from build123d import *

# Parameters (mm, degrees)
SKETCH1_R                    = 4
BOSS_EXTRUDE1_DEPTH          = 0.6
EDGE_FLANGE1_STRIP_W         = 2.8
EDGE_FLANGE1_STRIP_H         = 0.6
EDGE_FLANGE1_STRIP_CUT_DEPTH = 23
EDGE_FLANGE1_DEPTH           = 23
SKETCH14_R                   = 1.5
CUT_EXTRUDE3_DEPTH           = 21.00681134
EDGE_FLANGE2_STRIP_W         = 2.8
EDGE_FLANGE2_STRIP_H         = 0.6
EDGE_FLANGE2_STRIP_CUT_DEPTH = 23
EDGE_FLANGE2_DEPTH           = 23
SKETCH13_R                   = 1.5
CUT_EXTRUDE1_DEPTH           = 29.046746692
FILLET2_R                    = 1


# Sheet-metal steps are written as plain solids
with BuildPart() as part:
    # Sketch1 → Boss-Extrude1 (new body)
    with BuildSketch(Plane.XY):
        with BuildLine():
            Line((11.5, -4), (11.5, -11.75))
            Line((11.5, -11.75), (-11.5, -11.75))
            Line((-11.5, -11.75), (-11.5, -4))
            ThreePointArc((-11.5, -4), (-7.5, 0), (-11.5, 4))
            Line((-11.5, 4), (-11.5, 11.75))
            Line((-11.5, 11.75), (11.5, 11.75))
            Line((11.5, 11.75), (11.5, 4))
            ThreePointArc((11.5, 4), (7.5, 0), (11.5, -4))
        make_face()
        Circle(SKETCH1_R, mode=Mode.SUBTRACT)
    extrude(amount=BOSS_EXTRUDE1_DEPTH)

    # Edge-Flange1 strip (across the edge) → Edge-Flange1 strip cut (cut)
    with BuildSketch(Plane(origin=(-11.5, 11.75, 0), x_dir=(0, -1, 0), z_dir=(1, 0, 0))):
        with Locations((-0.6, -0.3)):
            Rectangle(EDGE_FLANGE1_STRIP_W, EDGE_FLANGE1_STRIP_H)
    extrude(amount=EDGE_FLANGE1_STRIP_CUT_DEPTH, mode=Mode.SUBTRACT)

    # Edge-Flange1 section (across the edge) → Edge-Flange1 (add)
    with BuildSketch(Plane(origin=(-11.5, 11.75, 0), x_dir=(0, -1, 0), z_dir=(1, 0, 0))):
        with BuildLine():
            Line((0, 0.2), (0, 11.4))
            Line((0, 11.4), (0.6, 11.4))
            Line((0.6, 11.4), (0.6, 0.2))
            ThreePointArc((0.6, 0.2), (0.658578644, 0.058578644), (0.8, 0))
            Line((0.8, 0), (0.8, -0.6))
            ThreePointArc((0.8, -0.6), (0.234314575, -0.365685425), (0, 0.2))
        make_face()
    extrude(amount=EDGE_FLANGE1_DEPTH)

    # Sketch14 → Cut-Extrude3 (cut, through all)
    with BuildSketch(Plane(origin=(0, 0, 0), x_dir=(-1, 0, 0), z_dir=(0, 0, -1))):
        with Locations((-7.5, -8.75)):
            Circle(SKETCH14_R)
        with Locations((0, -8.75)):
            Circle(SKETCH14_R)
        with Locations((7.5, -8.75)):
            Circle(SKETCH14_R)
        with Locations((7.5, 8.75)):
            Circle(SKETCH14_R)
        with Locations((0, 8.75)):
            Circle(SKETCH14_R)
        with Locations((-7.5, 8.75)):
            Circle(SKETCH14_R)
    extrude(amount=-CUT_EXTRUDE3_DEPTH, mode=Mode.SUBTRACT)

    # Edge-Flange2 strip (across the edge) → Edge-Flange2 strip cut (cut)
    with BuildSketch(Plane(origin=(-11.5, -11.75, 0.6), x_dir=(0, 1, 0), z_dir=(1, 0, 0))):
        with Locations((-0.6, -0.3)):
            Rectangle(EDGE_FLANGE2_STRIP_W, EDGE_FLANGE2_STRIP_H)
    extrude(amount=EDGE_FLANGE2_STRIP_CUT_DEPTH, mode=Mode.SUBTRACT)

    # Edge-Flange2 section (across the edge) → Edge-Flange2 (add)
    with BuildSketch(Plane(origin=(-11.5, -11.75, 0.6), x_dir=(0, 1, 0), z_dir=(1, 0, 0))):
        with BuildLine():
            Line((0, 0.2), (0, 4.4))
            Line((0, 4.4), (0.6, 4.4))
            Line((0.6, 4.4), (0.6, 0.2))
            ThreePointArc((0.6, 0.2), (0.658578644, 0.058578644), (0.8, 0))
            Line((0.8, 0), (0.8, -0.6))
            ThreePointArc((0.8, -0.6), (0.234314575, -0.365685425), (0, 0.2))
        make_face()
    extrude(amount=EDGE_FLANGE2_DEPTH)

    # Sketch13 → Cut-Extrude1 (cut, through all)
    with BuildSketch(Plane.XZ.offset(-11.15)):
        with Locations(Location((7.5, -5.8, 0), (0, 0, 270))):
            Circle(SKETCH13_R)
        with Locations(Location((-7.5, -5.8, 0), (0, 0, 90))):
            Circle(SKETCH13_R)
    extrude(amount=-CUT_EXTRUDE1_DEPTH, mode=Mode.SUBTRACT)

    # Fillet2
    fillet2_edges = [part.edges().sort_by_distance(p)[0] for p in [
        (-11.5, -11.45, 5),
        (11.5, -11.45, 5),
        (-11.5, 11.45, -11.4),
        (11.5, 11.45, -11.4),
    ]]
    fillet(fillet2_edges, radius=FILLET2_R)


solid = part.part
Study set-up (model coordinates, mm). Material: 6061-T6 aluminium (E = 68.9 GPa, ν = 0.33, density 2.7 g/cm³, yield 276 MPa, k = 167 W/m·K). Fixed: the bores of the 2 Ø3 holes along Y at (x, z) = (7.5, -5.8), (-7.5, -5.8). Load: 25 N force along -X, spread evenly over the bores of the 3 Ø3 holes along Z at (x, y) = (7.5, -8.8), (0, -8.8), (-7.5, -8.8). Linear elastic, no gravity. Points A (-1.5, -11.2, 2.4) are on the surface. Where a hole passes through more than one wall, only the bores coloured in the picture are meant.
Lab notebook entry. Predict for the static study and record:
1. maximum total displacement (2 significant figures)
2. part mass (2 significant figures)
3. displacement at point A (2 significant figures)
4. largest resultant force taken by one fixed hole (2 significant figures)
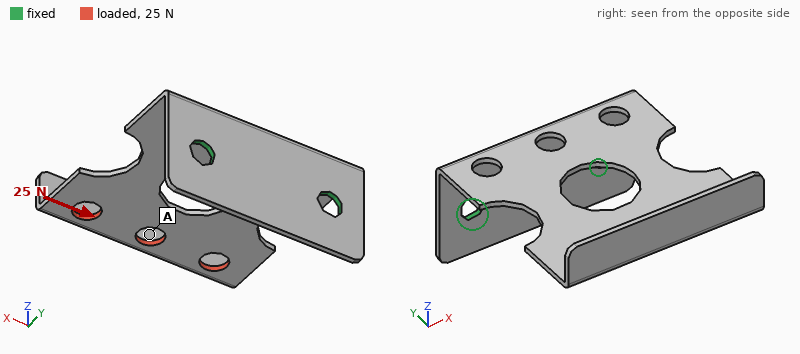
0.32 mm
1.2 g
0.21 mm
34 N
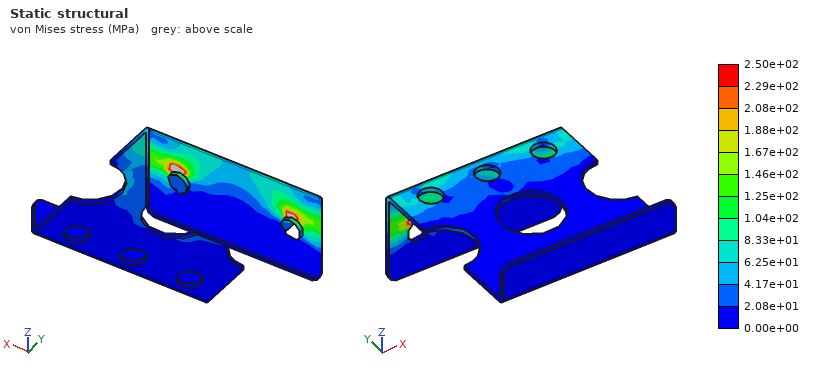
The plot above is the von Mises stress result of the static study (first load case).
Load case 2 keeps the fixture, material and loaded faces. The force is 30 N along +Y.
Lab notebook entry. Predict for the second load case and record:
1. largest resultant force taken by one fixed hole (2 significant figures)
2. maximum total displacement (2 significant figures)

15 N
0.34 mm
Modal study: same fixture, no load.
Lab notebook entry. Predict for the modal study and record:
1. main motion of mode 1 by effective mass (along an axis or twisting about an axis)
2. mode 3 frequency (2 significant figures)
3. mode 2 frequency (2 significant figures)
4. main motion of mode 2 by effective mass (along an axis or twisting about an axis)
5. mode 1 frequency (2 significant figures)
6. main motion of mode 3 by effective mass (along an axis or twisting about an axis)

along Z
2300 Hz
1500 Hz
twisting about Y
490 Hz
along X
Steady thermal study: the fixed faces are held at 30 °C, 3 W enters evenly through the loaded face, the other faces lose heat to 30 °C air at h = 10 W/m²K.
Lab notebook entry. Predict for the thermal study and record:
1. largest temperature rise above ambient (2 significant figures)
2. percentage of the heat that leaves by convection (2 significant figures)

52 K
13 %
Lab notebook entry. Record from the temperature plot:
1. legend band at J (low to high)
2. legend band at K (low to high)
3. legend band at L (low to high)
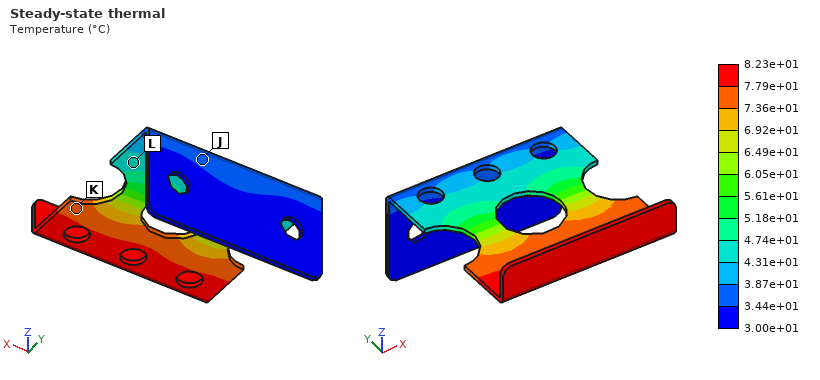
3.44e+01 to 3.87e+01 °C
7.36e+01 to 7.79e+01 °C
4.31e+01 to 4.74e+01 °C
